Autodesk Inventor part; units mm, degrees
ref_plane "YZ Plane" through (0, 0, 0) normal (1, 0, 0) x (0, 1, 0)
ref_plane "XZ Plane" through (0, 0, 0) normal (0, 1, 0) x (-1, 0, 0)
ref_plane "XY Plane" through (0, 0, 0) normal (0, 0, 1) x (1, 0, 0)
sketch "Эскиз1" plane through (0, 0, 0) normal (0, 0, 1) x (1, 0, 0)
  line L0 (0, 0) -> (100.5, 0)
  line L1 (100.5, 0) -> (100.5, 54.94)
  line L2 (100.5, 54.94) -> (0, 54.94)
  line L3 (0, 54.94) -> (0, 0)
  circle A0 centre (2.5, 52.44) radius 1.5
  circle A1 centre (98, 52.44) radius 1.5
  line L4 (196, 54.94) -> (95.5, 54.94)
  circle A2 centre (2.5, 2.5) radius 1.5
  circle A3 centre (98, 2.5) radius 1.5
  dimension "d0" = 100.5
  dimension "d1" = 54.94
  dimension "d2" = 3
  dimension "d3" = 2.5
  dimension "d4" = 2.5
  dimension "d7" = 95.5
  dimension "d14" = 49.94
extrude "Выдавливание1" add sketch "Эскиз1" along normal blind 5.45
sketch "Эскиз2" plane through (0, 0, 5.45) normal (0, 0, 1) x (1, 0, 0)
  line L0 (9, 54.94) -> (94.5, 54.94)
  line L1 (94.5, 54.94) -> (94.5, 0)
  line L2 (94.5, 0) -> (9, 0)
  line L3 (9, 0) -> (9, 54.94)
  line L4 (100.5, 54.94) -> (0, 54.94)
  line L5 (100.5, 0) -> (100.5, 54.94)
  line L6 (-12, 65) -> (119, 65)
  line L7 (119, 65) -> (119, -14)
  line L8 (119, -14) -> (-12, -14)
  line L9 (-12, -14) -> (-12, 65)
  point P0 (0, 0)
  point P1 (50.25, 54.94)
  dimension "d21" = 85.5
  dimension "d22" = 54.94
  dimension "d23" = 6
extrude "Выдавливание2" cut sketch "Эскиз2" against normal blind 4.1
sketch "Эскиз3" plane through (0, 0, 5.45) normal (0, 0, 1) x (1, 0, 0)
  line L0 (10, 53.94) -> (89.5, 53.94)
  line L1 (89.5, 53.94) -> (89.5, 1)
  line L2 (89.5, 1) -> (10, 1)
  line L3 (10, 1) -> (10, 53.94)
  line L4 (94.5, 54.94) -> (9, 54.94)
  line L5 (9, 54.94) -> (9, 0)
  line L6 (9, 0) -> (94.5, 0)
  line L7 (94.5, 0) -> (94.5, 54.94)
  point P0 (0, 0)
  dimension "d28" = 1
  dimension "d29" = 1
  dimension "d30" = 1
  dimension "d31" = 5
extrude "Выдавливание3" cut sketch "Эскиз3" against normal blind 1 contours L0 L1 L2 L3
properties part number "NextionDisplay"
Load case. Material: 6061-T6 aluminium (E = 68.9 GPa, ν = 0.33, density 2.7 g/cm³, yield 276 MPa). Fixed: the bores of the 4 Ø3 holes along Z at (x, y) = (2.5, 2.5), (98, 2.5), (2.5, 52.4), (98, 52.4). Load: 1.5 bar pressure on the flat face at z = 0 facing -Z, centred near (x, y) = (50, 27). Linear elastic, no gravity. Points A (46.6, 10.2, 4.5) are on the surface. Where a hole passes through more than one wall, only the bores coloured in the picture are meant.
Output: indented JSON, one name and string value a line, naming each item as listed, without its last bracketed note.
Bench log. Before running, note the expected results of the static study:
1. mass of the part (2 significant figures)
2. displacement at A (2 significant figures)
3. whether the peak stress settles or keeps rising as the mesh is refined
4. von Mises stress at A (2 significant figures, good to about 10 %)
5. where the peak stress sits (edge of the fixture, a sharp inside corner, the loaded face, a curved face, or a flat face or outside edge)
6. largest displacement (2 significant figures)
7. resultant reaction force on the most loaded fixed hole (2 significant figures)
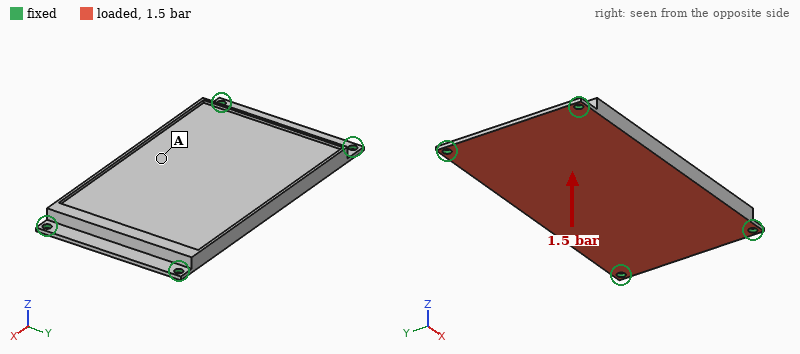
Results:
{
  "mass of the part": "61 g",
  "displacement at A": "0.18 mm",
  "whether the peak stress settles or keeps rising as the mesh is refined": "keeps rising",
  "von Mises stress at A": "34 MPa",
  "where the peak stress sits": "edge of the fixture",
  "largest displacement": "0.19 mm",
  "resultant reaction force on the most loaded fixed hole": "650 N"
}
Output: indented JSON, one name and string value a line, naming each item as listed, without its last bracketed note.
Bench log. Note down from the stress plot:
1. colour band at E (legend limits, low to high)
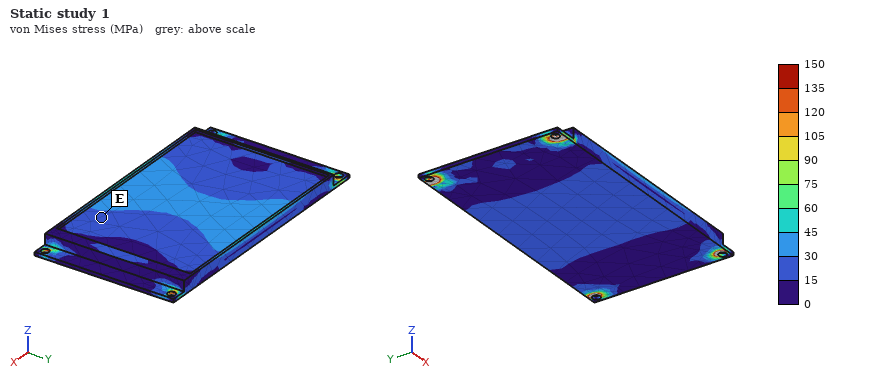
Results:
{
  "colour band at E": "15 to 30 MPa"
}
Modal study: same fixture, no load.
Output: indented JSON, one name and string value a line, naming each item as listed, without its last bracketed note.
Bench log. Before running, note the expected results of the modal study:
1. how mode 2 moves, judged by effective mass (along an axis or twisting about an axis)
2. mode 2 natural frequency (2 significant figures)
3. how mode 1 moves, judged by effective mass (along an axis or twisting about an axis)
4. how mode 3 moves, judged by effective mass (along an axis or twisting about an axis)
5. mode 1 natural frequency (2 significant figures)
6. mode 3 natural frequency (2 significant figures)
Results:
{
  "how mode 2 moves, judged by effective mass": "twisting about X",
  "mode 2 natural frequency": "2800 Hz",
  "how mode 1 moves, judged by effective mass": "along Z",
  "how mode 3 moves, judged by effective mass": "twisting about Y",
  "mode 1 natural frequency": "1500 Hz",
  "mode 3 natural frequency": "3800 Hz"
}
